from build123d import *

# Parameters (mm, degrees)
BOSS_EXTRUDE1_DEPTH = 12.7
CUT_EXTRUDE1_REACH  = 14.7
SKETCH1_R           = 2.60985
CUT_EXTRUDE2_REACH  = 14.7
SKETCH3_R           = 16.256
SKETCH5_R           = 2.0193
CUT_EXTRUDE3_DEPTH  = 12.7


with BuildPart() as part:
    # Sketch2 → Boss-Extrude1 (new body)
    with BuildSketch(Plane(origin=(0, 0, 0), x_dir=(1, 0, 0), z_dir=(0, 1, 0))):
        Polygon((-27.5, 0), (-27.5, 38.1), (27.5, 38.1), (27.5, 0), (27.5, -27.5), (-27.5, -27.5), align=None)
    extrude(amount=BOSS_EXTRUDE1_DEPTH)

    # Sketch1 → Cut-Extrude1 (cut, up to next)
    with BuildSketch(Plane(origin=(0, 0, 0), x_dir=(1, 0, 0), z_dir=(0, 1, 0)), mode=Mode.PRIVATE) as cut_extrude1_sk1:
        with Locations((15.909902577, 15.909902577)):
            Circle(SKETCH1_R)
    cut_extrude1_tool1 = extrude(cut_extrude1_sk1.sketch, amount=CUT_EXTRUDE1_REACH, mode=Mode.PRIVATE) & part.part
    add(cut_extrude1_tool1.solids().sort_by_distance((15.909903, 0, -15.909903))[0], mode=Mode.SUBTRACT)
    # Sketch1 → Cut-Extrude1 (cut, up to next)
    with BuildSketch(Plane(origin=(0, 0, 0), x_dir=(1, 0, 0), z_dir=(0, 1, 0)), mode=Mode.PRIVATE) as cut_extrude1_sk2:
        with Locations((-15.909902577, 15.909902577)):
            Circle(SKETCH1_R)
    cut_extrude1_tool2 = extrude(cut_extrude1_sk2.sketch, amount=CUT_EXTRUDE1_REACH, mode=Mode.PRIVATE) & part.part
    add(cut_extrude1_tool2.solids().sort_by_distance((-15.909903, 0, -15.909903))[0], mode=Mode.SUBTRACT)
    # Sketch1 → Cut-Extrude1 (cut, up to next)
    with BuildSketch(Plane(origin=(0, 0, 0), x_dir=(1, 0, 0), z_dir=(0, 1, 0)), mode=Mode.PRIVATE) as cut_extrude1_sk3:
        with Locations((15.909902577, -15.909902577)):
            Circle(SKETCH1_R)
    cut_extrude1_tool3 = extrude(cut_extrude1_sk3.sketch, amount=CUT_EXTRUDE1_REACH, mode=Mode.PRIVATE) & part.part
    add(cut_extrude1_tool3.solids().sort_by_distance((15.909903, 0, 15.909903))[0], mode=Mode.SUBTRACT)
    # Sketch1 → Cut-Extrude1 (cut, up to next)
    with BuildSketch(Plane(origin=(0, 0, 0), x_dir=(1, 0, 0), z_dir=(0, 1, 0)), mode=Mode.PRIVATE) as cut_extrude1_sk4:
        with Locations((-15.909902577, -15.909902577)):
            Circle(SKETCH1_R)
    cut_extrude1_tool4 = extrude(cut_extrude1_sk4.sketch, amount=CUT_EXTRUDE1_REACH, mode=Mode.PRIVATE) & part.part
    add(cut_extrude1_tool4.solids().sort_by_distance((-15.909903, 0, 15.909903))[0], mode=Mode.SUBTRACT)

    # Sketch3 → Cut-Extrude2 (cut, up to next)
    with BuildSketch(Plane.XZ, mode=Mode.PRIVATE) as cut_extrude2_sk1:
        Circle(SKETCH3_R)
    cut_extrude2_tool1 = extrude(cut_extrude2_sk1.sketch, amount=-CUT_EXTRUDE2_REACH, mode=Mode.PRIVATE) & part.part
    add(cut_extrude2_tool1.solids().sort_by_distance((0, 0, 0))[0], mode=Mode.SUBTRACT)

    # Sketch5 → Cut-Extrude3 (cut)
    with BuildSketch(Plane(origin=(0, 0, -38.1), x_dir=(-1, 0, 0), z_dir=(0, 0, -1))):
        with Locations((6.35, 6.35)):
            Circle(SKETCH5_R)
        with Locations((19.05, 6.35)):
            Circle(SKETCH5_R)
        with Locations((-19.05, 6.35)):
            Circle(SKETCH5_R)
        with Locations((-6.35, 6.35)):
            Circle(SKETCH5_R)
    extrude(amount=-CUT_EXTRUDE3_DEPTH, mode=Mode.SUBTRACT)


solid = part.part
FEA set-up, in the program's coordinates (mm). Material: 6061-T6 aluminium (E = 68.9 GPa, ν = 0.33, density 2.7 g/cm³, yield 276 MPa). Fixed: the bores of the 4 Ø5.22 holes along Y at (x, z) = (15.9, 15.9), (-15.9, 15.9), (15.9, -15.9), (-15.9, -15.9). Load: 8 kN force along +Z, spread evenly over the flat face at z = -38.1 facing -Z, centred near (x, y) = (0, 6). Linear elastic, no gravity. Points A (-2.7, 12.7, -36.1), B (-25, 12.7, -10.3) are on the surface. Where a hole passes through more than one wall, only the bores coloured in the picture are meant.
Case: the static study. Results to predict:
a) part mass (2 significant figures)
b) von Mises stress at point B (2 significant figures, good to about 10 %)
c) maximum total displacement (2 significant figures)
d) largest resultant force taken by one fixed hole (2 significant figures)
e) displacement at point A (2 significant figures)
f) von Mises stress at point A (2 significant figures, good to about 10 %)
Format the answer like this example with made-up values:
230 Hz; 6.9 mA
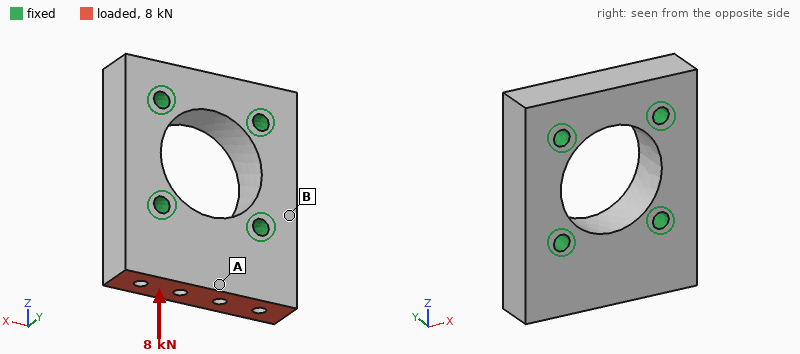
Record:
91 g; 5.4 MPa; 5.7 µm; 3.8 kN; 5.4 µm; 11 MPa
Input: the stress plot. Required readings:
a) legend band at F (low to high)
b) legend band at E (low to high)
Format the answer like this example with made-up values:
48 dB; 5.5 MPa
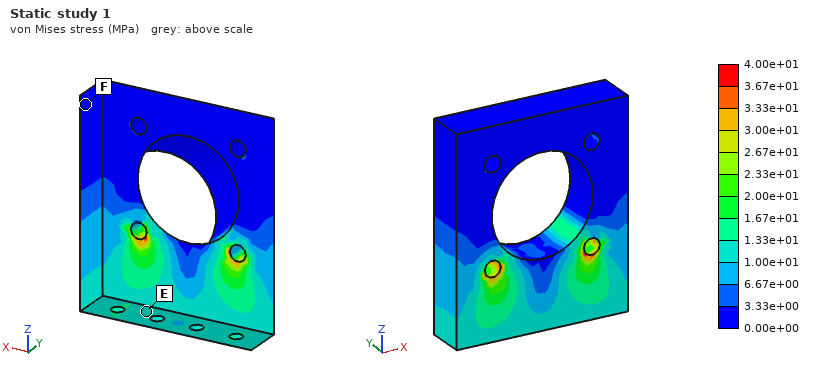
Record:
0.00e+00 to 3.33e+00 MPa; 1.00e+01 to 1.33e+01 MPa
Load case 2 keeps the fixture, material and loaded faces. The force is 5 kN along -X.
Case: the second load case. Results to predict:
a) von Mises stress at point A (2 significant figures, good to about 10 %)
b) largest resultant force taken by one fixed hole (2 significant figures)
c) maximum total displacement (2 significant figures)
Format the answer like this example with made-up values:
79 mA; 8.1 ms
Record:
18 MPa; 3.5 kN; 16 µm
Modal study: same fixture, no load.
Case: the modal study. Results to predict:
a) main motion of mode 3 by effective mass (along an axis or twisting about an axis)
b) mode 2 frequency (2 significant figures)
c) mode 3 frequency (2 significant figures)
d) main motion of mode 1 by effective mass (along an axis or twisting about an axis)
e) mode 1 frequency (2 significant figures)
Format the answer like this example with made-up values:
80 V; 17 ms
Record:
along X; 20 kHz; 26 kHz; along Y; 15 kHz
